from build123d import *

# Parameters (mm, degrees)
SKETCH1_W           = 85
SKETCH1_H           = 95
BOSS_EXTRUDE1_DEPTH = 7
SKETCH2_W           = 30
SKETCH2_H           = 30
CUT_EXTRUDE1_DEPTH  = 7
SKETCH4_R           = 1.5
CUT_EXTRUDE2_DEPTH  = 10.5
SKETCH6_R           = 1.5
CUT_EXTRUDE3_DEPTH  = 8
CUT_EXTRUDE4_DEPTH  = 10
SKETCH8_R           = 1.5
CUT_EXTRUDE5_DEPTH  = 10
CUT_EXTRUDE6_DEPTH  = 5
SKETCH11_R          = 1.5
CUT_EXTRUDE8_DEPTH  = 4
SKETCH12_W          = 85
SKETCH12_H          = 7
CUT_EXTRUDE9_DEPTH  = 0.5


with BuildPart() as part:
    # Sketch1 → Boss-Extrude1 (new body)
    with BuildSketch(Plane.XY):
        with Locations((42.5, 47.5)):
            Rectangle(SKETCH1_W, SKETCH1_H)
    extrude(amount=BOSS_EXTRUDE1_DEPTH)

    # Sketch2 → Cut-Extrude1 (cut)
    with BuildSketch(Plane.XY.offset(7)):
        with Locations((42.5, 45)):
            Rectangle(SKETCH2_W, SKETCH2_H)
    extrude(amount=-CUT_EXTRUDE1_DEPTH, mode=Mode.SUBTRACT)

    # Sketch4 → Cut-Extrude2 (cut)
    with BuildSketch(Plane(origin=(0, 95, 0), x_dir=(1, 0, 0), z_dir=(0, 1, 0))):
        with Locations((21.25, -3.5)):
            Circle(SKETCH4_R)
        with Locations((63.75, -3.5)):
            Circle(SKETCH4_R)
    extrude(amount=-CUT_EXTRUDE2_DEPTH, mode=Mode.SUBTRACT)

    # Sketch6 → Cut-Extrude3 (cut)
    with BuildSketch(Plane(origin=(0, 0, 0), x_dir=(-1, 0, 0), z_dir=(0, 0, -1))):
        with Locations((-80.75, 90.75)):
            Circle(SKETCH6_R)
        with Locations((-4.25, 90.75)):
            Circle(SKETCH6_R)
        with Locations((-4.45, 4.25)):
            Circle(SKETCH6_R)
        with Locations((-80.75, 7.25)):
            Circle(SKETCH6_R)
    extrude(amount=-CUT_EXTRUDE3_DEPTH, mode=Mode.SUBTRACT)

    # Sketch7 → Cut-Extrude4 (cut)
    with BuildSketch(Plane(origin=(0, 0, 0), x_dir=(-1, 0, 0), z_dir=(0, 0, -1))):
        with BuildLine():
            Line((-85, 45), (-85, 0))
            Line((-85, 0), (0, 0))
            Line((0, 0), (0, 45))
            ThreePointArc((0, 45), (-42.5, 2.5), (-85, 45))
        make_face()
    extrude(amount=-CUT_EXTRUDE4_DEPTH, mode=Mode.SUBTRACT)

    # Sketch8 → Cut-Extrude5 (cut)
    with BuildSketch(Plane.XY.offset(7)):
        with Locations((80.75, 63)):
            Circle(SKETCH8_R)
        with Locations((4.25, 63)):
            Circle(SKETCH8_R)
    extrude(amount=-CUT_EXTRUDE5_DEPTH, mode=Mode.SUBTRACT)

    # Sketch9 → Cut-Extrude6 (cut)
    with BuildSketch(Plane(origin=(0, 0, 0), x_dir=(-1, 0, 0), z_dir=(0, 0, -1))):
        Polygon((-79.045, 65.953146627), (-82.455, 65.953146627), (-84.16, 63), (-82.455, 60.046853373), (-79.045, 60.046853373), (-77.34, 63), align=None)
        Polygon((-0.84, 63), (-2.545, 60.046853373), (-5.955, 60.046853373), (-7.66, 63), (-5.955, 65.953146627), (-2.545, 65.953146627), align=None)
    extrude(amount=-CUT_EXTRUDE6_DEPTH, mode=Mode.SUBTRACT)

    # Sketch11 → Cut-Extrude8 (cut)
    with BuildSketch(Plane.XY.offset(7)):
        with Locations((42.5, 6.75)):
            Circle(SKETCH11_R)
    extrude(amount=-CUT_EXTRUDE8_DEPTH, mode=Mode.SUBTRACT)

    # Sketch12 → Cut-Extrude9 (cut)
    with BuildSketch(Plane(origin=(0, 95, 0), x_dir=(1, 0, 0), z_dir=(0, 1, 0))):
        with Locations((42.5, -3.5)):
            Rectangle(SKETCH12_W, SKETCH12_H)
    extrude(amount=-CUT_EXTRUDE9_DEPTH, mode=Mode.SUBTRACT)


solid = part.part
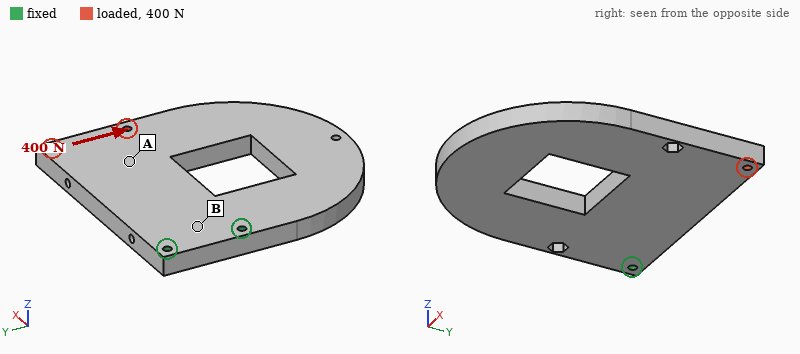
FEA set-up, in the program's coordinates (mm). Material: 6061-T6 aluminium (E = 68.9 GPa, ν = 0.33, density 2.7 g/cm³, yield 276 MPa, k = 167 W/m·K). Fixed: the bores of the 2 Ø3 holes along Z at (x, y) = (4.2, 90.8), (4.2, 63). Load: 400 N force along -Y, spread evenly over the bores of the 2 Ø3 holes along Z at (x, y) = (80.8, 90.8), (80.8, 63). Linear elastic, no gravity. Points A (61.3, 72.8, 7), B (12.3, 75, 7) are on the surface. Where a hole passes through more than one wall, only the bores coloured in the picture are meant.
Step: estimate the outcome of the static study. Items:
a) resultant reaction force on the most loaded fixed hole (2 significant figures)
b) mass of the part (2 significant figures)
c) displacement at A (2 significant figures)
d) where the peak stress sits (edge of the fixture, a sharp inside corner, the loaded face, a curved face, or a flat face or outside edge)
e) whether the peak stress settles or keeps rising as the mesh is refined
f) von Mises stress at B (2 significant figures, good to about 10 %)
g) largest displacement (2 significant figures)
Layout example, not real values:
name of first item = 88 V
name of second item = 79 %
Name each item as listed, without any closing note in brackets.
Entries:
resultant reaction force on the most loaded fixed hole = 1.1 kN
mass of the part = 110 g
displacement at A = 0.058 mm
where the peak stress sits = edge of the fixture
whether the peak stress settles or keeps rising as the mesh is refined = keeps rising
von Mises stress at B = 12 MPa
largest displacement = 0.10 mm
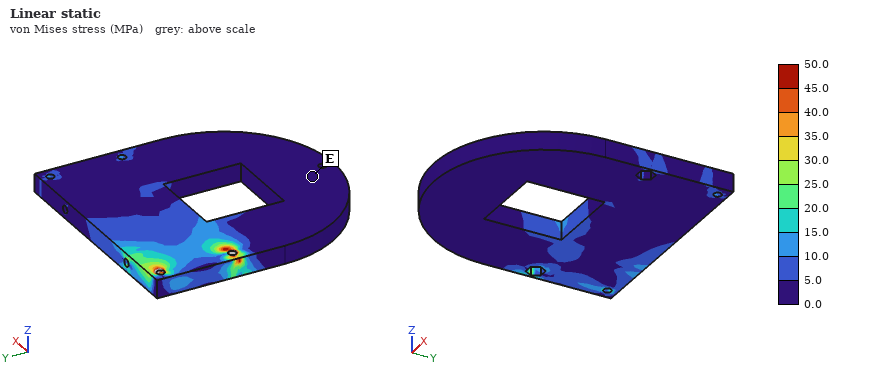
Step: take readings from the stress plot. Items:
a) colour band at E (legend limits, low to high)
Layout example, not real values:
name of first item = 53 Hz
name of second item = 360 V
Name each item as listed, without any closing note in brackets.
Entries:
colour band at E = 0.0 to 5.0 MPa
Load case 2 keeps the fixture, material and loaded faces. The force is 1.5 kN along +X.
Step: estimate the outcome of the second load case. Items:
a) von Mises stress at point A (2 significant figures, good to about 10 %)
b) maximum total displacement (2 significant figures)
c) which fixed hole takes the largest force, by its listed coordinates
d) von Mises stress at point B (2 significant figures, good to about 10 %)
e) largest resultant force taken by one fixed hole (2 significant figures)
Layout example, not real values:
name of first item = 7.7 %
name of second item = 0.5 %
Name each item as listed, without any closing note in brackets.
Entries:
von Mises stress at point A = 5.0 MPa
maximum total displacement = 32 µm
which fixed hole takes the largest force, by its listed coordinates = (4.2, 90.8)
von Mises stress at point B = 3.8 MPa
largest resultant force taken by one fixed hole = 1.2 kN
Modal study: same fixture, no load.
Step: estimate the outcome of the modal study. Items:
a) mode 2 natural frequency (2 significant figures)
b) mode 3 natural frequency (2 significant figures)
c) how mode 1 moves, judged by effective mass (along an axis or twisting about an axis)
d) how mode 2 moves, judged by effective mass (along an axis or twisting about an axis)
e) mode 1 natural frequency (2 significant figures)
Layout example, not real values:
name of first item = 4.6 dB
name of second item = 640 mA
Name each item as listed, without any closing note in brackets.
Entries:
mode 2 natural frequency = 1100 Hz
mode 3 natural frequency = 2000 Hz
how mode 1 moves, judged by effective mass = along Z
how mode 2 moves, judged by effective mass = twisting about X
mode 1 natural frequency = 450 Hz
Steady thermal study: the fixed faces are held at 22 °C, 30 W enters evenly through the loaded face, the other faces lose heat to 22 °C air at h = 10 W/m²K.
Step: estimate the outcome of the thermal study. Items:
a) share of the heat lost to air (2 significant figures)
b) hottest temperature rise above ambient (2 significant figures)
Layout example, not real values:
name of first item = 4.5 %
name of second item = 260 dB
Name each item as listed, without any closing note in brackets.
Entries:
share of the heat lost to air = 12 %
hottest temperature rise above ambient = 60 K
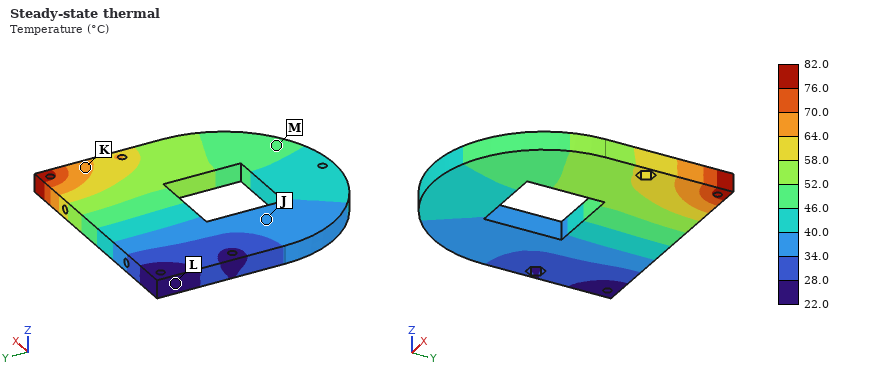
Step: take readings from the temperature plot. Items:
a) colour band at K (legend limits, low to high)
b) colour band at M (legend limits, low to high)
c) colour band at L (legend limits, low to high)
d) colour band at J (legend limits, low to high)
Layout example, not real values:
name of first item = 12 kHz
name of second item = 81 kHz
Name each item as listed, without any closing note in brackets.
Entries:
colour band at K = 64.0 to 70.0 °C
colour band at M = 46.0 to 52.0 °C
colour band at L = 22.0 to 28.0 °C
colour band at J = 34.0 to 40.0 °C
